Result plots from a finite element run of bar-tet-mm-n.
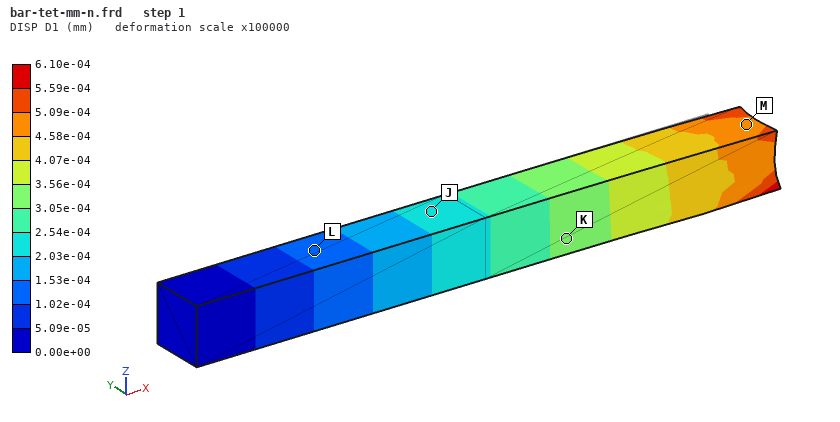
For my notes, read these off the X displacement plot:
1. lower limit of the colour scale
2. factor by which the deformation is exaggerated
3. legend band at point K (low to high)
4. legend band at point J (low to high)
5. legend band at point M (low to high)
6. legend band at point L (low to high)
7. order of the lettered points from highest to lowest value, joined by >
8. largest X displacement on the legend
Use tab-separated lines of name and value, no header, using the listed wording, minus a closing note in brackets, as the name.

lower limit of the colour scale	0.00e+00 mm
factor by which the deformation is exaggerated	100000
legend band at point K	3.05e-04 to 3.56e-04 mm
legend band at point J	2.03e-04 to 2.54e-04 mm
legend band at point M	4.58e-04 to 5.09e-04 mm
legend band at point L	1.02e-04 to 1.53e-04 mm
order of the lettered points from highest to lowest value, joined by >	M > K > J > L
largest X displacement on the legend	6.10e-04 mm
